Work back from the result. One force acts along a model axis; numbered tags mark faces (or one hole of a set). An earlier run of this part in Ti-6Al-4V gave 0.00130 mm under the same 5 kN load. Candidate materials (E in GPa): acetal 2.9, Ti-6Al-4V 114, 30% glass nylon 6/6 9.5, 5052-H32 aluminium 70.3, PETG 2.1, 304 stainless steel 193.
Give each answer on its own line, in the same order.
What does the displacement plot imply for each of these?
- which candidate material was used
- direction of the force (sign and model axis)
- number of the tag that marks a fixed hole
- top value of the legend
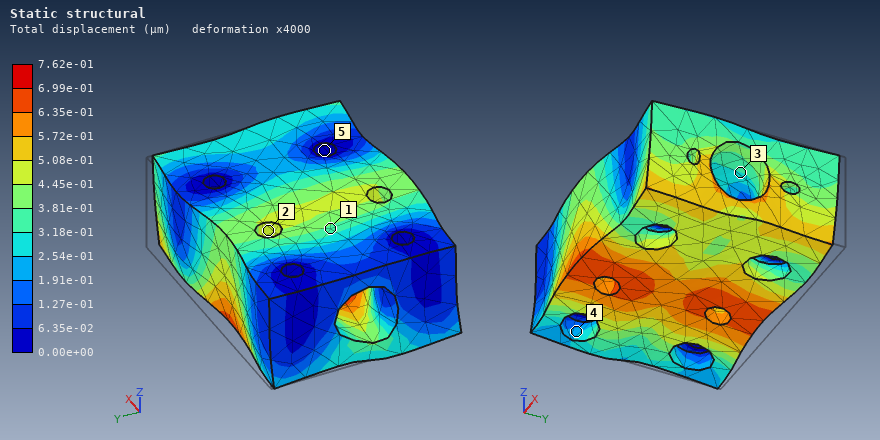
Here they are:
304 stainless steel
-Y
5
7.62e-01 µm
